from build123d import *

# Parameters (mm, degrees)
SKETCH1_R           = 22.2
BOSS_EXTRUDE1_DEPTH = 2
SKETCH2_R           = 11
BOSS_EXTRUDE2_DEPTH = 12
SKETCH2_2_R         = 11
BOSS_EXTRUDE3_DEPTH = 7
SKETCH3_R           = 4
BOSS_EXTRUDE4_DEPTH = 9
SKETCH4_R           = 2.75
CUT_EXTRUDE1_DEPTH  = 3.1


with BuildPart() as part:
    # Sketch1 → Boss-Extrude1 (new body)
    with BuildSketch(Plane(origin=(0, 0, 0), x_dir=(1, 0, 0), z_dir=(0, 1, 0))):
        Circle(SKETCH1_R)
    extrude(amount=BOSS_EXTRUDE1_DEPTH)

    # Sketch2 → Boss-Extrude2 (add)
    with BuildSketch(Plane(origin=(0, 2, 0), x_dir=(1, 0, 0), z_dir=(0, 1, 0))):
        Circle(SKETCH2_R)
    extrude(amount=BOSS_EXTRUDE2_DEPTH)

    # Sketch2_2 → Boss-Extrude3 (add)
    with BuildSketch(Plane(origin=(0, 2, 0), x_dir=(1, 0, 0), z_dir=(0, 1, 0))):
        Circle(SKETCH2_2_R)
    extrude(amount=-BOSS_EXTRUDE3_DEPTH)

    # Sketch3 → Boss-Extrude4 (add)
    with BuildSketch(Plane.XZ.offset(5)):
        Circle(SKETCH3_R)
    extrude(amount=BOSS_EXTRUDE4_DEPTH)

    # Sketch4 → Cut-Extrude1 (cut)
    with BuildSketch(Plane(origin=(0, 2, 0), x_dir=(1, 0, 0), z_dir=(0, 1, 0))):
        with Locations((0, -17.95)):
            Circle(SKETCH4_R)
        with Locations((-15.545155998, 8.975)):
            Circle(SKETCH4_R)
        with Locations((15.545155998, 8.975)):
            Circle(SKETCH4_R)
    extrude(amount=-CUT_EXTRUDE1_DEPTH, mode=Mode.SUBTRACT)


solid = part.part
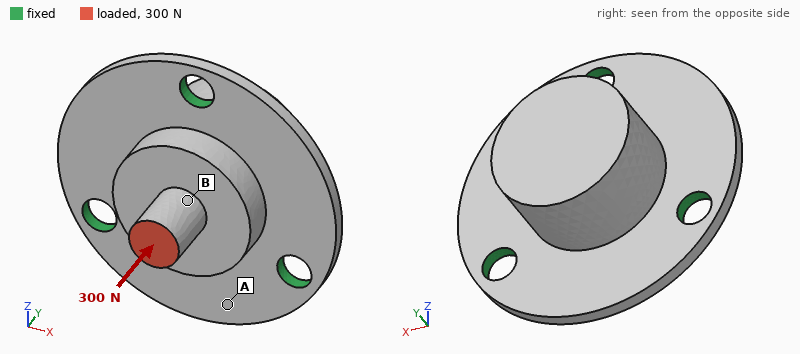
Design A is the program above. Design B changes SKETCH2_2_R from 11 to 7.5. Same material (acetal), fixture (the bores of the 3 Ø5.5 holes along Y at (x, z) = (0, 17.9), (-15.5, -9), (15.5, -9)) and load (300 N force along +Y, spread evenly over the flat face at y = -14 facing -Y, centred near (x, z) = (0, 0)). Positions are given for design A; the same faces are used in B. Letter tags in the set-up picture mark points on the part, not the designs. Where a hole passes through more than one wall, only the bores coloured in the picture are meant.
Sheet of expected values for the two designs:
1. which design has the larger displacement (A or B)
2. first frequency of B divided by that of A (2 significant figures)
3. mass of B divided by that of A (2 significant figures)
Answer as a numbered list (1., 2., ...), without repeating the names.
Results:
1. B
2. 1.00
3. 0.90
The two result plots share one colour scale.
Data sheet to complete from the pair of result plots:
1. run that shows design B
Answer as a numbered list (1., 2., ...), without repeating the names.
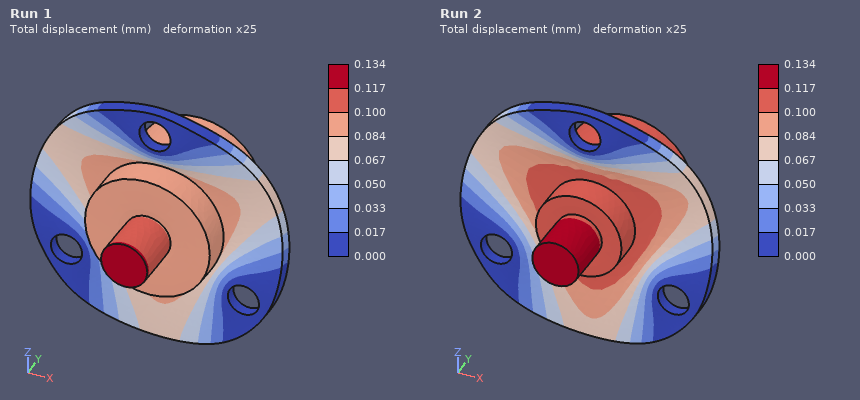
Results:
1. Run 2
